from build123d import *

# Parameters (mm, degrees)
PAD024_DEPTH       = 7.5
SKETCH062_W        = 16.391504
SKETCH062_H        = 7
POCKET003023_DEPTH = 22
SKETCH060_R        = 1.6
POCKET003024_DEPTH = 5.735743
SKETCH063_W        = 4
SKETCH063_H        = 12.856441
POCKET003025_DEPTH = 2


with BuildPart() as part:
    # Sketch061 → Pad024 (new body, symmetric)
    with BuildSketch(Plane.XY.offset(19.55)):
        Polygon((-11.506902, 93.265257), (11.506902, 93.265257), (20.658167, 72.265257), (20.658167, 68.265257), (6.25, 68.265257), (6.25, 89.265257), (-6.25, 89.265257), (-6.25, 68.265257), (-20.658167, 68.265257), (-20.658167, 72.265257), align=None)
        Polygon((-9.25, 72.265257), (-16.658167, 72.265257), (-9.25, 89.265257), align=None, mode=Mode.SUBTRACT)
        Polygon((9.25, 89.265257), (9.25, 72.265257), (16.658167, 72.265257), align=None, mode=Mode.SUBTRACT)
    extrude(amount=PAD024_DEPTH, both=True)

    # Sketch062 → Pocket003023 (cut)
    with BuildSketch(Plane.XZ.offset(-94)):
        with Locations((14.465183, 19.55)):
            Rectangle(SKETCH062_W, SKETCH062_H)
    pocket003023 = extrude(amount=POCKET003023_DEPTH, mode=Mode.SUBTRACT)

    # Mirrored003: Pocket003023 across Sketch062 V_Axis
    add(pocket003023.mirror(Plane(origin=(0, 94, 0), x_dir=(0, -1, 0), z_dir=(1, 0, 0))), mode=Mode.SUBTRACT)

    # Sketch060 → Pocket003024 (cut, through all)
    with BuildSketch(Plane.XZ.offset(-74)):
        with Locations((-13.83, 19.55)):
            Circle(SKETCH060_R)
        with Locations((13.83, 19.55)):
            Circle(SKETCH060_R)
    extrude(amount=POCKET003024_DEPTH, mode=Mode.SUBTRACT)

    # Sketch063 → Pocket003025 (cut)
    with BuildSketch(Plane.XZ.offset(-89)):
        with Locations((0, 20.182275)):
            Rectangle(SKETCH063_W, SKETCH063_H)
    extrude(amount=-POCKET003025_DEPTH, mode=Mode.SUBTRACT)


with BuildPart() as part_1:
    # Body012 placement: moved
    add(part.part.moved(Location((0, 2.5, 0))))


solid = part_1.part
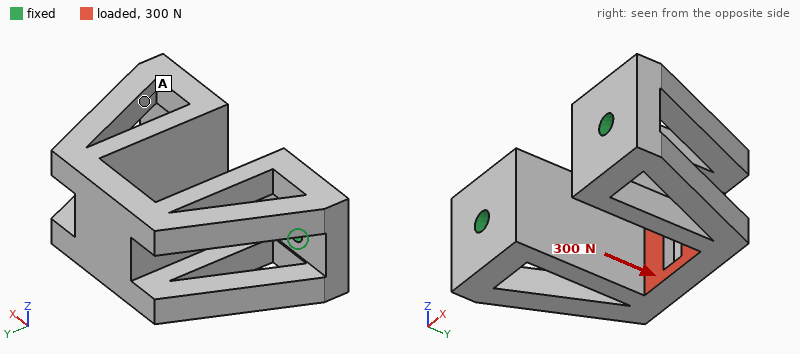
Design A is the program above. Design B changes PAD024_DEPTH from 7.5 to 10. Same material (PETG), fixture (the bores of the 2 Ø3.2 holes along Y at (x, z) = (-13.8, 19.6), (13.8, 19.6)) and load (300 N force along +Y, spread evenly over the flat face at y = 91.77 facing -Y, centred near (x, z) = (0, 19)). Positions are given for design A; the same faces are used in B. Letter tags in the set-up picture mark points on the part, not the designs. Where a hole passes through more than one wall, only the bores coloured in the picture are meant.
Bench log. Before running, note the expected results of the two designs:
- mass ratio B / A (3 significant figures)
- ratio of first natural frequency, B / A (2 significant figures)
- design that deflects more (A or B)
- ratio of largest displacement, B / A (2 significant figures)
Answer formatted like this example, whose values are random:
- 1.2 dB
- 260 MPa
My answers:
- 1.49
- 0.93
- A
- 0.72
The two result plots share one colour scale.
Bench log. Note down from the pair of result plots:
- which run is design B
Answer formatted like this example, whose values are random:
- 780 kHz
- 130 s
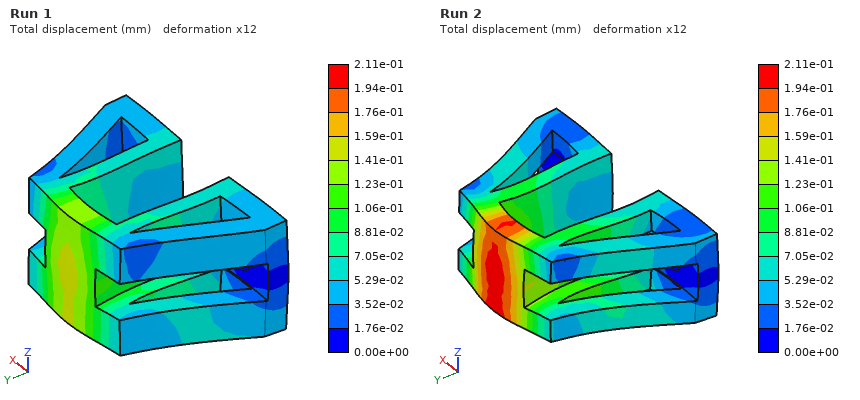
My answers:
- Run 1
